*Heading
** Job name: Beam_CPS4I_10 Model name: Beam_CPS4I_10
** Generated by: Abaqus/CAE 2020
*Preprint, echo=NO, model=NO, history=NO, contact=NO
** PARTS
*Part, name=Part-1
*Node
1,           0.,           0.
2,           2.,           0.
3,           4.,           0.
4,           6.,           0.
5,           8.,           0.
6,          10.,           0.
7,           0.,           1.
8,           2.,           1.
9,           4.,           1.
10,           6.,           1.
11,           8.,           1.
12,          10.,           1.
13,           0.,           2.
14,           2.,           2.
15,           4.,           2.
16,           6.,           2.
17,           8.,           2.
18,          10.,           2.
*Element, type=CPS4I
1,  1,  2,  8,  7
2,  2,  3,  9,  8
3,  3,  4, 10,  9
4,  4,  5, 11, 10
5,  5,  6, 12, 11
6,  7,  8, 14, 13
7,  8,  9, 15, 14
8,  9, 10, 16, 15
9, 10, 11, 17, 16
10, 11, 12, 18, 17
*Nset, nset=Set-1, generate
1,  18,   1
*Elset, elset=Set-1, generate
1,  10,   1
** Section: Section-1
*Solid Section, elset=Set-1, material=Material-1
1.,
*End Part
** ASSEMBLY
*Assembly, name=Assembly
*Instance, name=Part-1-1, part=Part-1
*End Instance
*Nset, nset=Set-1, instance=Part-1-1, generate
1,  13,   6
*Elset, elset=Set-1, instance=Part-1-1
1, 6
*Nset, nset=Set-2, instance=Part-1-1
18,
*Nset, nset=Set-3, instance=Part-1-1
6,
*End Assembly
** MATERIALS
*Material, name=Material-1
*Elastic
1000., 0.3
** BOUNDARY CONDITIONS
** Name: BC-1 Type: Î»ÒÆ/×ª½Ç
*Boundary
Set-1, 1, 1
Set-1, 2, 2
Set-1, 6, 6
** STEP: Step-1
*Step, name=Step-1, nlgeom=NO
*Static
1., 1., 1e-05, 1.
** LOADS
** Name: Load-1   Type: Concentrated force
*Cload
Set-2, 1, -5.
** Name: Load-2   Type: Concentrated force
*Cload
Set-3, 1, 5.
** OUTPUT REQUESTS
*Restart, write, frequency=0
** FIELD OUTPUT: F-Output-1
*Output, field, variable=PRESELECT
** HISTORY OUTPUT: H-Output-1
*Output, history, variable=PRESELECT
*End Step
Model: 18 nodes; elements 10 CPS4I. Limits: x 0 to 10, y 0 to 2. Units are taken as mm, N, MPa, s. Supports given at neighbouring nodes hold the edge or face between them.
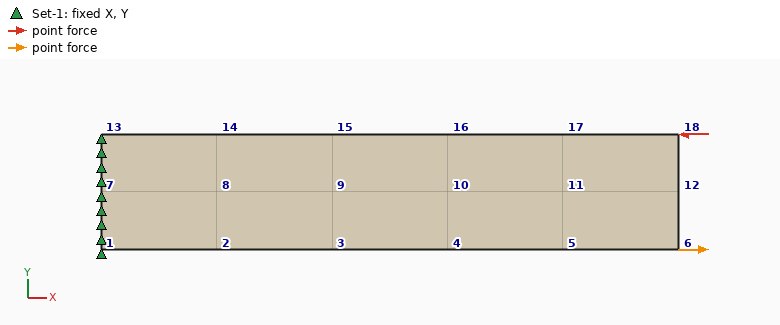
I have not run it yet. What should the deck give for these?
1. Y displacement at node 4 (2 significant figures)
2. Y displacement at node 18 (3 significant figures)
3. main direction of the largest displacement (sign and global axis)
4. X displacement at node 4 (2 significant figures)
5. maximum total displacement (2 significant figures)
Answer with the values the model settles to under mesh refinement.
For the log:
0.27 mm
0.755 mm
+Y
0.089 mm
0.77 mm
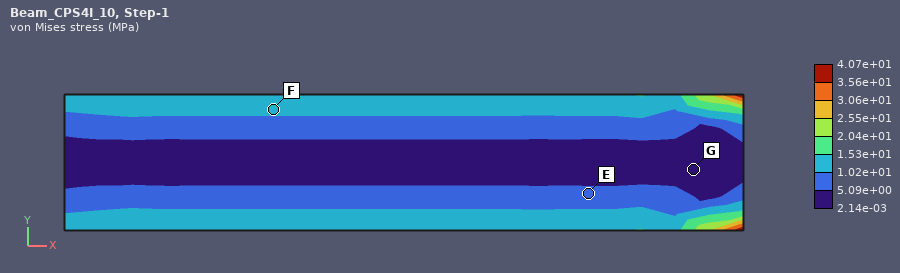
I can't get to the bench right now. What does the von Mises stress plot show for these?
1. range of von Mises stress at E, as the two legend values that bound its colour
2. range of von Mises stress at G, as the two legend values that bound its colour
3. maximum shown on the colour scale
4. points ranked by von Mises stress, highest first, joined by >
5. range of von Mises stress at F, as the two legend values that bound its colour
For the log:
5.09e+00 to 1.02e+01 MPa
2.14e-03 to 5.09e+00 MPa
4.07e+01 MPa
F > E > G
1.02e+01 to 1.53e+01 MPa
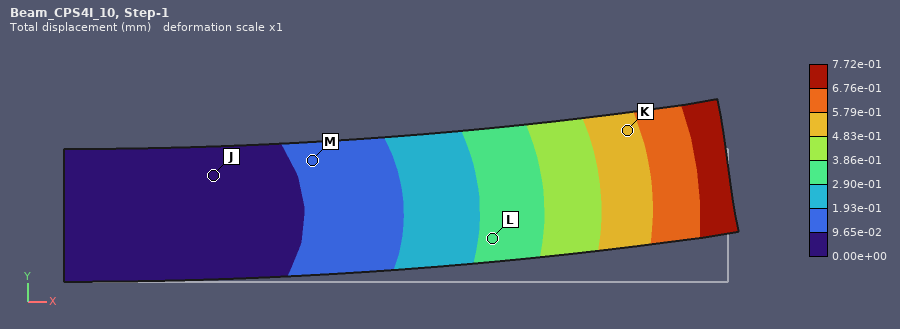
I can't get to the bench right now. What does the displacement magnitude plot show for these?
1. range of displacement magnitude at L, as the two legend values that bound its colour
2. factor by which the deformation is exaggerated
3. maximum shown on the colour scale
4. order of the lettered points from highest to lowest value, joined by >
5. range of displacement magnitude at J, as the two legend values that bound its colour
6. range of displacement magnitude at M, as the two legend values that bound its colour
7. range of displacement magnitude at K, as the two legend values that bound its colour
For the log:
2.90e-01 to 3.86e-01 mm
1
7.72e-01 mm
K > L > M > J
0.00e+00 to 9.65e-02 mm
9.65e-02 to 1.93e-01 mm
4.83e-01 to 5.79e-01 mm
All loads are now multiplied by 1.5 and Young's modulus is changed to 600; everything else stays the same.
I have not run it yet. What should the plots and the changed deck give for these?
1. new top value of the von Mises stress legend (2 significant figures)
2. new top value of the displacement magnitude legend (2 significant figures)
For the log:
61 MPa
1.9 mm
